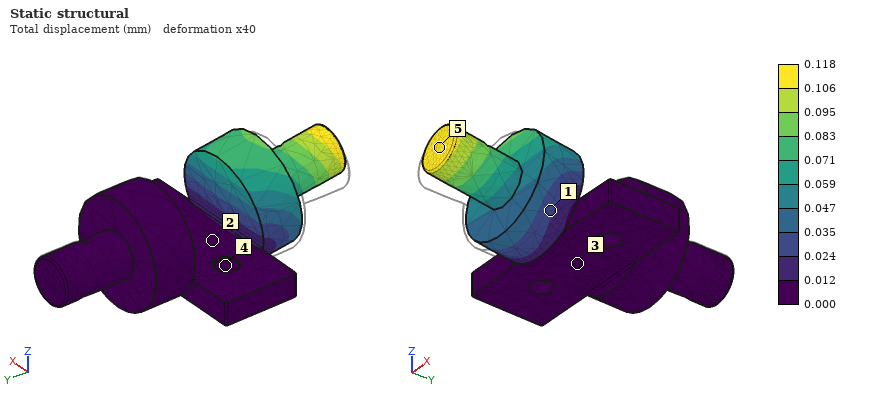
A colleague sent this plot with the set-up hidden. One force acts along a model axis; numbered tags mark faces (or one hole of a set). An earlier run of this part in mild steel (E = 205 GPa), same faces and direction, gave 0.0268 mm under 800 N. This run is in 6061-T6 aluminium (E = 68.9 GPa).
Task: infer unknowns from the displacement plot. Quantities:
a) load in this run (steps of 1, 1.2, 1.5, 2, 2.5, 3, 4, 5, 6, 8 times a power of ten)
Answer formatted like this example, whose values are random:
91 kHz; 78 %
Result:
1.2 kN
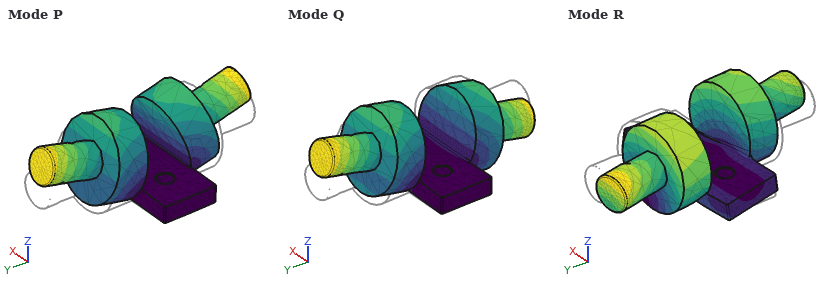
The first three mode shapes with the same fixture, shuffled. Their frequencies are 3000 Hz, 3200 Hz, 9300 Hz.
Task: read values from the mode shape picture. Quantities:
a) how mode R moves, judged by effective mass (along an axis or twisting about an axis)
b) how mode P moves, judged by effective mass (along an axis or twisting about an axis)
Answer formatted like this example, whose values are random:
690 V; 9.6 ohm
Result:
twisting about Z; along Z
